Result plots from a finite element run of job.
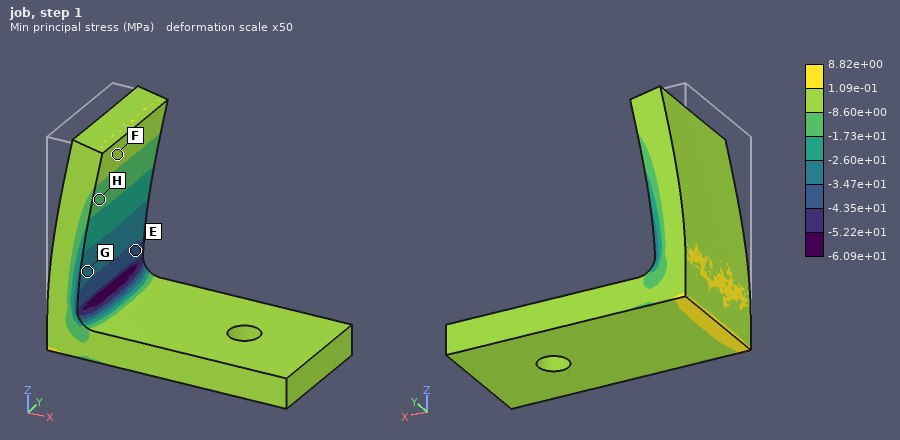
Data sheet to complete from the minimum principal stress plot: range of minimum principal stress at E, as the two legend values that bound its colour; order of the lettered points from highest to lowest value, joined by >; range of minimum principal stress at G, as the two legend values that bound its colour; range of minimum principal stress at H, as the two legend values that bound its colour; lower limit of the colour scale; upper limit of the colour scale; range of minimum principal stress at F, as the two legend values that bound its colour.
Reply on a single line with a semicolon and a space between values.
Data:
-4.35e+01 to -3.47e+01 MPa; F > H > G > E; -3.47e+01 to -2.60e+01 MPa; -1.73e+01 to -8.60e+00 MPa; -6.09e+01 MPa; 8.82e+00 MPa; -8.60e+00 to 1.09e-01 MPa
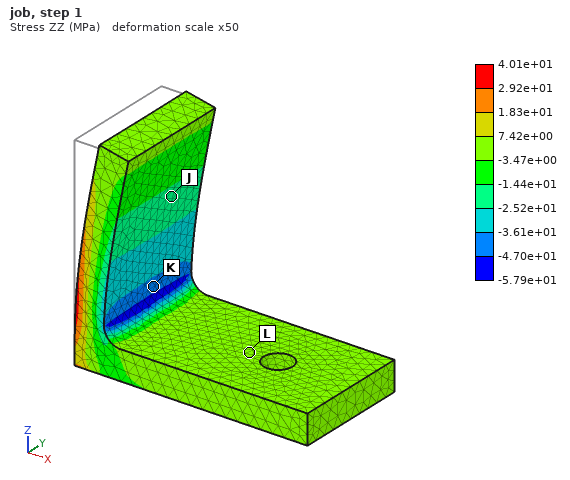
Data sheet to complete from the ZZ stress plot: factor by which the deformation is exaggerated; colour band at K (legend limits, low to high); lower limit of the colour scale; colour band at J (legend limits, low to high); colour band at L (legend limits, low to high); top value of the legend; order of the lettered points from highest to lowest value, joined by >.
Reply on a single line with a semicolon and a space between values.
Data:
50; -4.70e+01 to -3.61e+01 MPa; -5.79e+01 MPa; -2.52e+01 to -1.44e+01 MPa; -3.47e+00 to 7.42e+00 MPa; 4.01e+01 MPa; L > J > K
